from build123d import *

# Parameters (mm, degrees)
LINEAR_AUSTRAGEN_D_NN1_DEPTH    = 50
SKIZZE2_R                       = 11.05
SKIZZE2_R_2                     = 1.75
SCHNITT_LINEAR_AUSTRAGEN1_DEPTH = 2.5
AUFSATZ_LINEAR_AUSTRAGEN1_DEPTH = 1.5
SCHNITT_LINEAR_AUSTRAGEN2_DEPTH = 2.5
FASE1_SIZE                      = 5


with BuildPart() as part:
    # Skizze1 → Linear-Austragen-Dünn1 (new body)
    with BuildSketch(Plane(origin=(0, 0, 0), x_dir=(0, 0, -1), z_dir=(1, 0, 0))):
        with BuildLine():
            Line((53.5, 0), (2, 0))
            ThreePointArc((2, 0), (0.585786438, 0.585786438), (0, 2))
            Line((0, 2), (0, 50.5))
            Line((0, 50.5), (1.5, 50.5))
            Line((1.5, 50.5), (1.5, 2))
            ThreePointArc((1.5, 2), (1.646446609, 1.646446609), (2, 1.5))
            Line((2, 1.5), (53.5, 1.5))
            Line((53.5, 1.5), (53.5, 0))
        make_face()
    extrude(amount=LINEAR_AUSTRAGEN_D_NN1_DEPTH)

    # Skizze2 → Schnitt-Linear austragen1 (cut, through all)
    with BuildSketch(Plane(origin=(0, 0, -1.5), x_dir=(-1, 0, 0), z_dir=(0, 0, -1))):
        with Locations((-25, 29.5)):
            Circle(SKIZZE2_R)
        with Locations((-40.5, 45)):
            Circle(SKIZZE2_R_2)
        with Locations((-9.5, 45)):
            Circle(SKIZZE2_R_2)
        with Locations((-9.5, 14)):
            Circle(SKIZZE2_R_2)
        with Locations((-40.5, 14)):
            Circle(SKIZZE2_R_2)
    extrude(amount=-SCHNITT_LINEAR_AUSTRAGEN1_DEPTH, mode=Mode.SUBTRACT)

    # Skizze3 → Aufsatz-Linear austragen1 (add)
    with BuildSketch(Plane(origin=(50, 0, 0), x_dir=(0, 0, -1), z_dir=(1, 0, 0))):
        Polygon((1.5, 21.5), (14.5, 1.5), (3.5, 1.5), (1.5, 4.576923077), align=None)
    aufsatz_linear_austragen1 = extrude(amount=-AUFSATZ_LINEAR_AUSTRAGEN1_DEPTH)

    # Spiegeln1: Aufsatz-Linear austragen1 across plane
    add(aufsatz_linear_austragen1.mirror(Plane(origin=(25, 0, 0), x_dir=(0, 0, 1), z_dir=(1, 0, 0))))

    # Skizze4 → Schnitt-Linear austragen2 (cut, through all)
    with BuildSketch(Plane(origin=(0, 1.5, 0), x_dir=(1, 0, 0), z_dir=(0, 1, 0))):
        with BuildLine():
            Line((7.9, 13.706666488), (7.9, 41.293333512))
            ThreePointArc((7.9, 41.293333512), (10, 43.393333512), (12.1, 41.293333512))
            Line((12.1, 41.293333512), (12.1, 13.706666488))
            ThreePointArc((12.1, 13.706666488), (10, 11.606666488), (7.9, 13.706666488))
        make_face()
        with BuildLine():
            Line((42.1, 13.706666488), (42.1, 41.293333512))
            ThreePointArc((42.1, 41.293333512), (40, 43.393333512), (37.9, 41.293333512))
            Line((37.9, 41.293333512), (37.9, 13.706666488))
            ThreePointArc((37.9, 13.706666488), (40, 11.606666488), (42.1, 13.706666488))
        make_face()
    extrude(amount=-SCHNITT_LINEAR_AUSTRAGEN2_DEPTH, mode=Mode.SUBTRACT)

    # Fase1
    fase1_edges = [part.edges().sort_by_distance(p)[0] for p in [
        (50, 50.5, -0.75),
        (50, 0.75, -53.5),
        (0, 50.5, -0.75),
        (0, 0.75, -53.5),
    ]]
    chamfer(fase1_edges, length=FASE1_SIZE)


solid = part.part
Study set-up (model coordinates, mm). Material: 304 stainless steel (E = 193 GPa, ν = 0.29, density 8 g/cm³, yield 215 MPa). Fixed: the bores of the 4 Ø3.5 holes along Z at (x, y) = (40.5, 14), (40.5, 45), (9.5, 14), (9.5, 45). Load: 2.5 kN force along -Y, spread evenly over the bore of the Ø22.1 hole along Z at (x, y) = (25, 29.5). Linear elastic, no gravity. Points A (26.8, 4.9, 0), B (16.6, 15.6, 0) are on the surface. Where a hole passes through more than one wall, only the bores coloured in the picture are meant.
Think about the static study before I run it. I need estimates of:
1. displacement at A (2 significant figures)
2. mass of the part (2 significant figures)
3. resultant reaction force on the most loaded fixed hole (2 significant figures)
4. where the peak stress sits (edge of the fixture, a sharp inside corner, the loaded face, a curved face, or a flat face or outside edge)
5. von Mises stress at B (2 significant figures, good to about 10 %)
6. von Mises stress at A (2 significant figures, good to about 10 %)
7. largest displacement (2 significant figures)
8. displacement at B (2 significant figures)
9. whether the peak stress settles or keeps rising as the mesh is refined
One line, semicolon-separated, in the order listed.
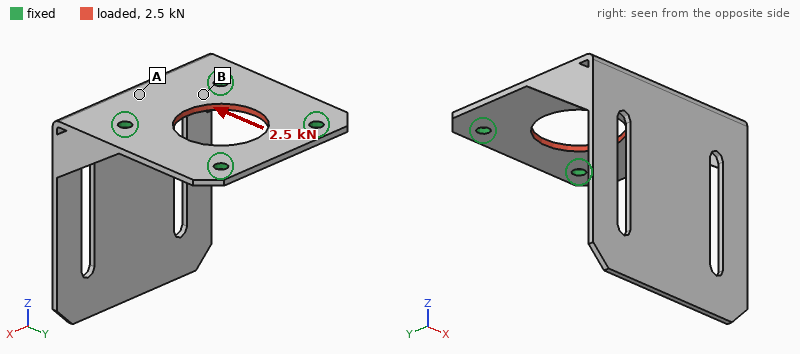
2.1 µm; 55 g; 650 N; edge of the fixture; 21 MPa; 10 MPa; 5.3 µm; 1.7 µm; keeps rising
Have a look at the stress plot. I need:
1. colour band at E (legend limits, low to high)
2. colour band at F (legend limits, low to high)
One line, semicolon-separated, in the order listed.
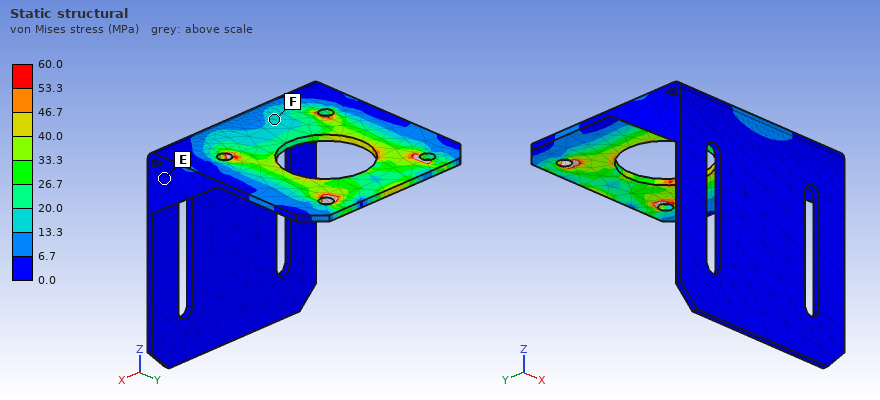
0.0 to 6.7 MPa; 13.3 to 20.0 MPa
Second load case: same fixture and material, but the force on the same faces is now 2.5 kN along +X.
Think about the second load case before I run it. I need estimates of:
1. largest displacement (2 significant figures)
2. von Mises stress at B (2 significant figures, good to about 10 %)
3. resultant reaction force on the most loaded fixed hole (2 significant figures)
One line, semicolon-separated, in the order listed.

4.0 µm; 32 MPa; 650 N
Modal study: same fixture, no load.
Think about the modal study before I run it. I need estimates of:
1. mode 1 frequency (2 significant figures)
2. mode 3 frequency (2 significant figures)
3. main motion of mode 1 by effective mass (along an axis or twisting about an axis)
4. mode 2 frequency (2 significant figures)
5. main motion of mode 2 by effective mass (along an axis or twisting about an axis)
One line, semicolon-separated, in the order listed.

450 Hz; 1600 Hz; along Y; 1100 Hz; along X
